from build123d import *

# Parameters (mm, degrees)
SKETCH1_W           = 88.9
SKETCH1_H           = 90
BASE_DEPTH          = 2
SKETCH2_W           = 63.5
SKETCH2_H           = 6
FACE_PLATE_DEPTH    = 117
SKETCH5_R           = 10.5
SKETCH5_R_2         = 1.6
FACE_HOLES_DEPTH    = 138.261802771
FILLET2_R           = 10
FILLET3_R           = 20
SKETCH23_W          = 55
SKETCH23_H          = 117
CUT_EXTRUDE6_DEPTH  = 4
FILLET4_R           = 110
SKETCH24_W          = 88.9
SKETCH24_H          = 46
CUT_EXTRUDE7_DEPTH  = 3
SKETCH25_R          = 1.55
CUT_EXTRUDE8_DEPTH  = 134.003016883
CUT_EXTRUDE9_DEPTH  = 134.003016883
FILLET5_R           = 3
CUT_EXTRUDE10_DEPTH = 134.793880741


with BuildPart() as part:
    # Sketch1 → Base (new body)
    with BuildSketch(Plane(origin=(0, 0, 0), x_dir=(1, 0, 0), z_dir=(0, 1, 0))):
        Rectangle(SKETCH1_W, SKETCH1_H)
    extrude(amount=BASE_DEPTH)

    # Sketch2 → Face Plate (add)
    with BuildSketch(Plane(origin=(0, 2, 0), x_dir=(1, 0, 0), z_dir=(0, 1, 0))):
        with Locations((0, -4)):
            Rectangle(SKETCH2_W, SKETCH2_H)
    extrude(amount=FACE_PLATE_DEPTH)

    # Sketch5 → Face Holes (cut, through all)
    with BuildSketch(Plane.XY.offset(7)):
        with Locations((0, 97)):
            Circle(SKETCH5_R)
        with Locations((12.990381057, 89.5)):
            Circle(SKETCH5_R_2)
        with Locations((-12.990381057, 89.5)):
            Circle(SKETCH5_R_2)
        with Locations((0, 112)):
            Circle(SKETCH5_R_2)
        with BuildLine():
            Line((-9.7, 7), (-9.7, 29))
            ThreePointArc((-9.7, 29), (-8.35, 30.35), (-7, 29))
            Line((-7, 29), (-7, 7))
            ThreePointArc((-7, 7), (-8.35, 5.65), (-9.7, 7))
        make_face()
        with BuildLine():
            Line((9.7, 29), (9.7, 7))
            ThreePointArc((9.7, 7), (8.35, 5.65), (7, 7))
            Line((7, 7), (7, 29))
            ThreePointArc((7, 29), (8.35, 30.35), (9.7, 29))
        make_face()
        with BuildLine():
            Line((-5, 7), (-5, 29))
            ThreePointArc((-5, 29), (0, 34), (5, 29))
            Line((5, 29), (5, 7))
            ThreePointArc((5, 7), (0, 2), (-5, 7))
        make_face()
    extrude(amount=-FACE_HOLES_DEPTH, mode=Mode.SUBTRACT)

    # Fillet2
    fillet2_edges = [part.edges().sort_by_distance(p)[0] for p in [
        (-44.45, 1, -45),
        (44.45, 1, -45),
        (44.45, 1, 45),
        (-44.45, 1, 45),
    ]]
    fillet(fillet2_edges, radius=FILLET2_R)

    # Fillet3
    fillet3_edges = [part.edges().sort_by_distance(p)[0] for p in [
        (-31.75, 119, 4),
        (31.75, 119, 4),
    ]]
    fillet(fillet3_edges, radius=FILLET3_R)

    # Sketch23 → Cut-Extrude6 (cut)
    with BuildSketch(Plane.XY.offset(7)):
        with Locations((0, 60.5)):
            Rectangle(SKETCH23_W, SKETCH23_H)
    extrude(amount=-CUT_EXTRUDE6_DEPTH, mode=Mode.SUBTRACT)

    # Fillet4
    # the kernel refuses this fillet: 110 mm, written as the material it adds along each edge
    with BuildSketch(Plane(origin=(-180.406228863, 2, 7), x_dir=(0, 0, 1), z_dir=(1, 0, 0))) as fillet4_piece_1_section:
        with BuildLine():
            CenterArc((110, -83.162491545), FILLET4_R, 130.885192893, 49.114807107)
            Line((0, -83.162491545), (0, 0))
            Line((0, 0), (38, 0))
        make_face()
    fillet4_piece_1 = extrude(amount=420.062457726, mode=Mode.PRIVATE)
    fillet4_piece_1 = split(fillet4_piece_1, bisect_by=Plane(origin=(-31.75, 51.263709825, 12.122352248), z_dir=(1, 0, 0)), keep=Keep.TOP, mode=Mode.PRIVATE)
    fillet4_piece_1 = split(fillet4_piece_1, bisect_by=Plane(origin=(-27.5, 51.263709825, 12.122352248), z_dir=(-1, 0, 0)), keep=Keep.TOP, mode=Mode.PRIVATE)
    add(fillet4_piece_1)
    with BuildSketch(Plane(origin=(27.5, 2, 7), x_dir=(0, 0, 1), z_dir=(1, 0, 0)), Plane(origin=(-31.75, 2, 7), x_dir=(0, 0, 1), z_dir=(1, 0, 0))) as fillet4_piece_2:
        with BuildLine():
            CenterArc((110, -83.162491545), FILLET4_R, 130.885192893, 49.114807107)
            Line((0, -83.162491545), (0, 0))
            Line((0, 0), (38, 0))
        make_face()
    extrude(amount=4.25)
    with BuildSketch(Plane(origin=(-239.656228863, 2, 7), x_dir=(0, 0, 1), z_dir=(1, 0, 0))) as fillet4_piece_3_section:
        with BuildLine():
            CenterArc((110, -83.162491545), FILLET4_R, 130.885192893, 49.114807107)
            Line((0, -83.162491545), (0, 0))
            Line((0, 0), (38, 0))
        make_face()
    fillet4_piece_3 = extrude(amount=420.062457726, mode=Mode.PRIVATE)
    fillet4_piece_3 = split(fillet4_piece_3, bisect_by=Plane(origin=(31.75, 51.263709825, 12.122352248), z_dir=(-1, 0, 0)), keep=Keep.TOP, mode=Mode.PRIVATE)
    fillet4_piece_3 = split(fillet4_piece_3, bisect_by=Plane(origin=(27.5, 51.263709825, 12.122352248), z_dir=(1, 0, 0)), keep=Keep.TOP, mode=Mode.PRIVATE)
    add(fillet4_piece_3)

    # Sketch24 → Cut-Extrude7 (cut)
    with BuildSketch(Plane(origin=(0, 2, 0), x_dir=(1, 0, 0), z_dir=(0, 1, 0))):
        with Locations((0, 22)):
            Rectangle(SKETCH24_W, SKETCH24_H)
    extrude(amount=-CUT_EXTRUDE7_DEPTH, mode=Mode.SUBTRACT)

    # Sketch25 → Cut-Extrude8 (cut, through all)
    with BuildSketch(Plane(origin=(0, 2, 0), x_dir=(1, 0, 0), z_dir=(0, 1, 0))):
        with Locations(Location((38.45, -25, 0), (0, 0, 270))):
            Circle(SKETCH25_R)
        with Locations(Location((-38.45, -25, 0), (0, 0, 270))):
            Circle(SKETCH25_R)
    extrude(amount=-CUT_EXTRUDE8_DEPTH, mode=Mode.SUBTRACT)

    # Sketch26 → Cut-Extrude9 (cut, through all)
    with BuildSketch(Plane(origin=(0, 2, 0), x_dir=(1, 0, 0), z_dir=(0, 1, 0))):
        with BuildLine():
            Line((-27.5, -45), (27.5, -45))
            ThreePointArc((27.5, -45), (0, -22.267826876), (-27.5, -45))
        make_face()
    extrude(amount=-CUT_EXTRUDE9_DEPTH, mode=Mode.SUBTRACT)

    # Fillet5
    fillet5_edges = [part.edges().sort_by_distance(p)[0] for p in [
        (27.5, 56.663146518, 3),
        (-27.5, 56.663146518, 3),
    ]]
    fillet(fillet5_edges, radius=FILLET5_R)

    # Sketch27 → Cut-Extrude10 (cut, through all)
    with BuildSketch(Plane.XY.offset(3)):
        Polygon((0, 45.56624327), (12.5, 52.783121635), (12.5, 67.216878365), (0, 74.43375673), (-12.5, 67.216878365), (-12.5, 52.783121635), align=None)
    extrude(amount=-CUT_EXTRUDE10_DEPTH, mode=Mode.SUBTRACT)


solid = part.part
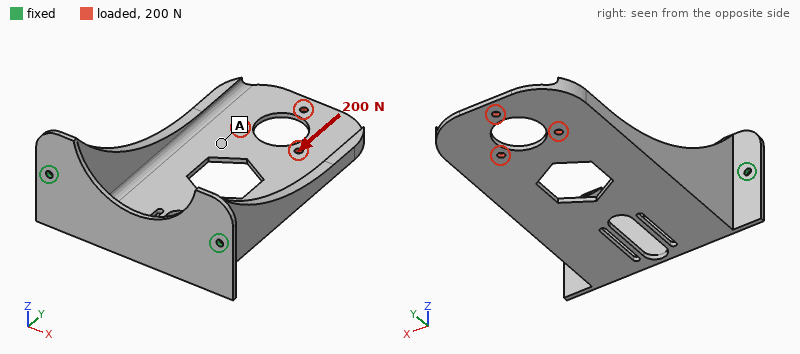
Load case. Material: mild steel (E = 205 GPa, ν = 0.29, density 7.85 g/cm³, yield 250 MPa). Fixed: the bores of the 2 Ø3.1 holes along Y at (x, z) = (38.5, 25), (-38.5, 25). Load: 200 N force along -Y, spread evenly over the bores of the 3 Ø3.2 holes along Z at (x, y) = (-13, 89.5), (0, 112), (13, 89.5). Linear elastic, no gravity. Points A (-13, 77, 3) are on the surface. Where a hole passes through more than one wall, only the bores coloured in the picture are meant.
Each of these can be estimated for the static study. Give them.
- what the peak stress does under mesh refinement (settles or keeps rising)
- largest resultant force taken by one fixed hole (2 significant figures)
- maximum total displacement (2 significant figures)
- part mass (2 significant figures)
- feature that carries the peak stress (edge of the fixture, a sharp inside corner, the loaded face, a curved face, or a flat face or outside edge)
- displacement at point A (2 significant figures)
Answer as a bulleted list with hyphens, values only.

- keeps rising
- 100 N
- 0.30 mm
- 230 g
- edge of the fixture
- 0.20 mm
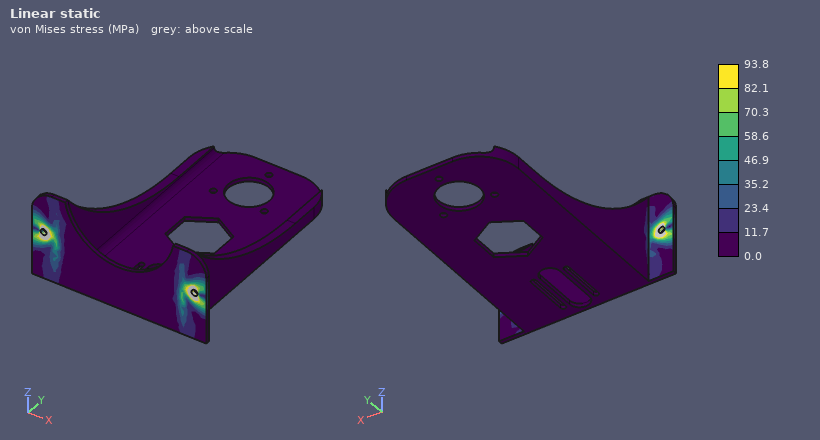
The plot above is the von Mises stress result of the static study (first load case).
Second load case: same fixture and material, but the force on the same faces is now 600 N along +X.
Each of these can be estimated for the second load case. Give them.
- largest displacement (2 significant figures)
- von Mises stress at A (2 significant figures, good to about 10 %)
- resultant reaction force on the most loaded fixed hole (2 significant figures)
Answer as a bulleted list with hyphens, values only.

- 0.58 mm
- 59 MPa
- 850 N
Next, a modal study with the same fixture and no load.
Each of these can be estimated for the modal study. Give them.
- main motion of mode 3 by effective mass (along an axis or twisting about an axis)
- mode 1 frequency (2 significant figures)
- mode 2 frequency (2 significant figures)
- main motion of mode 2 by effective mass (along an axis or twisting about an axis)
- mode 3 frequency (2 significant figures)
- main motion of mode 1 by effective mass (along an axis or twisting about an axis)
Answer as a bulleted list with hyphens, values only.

- along Y
- 260 Hz
- 570 Hz
- along X
- 1700 Hz
- along Z
